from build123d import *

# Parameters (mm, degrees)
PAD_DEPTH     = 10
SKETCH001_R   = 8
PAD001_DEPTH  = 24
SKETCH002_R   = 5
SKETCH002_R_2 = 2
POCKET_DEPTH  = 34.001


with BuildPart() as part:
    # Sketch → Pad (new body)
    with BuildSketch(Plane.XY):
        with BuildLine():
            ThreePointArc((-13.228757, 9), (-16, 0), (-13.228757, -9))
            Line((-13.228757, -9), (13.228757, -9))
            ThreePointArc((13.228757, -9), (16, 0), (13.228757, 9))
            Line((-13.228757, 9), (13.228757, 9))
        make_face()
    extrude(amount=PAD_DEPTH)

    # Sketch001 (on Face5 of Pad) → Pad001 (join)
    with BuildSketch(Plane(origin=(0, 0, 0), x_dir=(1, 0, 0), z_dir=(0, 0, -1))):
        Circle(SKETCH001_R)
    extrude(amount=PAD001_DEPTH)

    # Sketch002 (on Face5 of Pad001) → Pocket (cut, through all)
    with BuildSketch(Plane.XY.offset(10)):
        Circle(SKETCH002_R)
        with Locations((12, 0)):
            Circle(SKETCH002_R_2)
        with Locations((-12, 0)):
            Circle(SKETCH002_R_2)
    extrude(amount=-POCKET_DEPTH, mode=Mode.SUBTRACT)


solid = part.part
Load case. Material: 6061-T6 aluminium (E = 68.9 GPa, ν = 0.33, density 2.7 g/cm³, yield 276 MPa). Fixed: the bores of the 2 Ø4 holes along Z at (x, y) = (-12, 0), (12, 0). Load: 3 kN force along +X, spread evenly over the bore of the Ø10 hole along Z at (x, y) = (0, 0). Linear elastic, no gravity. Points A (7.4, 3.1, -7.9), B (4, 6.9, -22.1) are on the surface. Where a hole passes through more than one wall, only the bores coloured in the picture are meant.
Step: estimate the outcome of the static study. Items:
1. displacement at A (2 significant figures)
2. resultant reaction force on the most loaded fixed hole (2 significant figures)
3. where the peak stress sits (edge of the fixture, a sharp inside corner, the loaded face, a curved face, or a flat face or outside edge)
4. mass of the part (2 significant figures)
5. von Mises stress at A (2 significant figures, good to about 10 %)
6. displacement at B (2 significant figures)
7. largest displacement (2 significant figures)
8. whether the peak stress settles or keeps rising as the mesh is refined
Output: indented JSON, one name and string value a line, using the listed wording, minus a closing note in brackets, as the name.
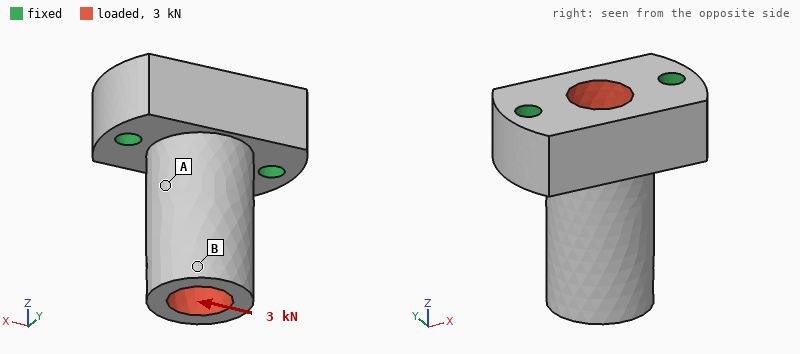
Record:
{
  "displacement at A": "21 µm",
  "resultant reaction force on the most loaded fixed hole": "2.3 kN",
  "where the peak stress sits": "a sharp inside corner",
  "mass of the part": "20 g",
  "von Mises stress at A": "29 MPa",
  "displacement at B": "46 µm",
  "largest displacement": "51 µm",
  "whether the peak stress settles or keeps rising as the mesh is refined": "keeps rising"
}
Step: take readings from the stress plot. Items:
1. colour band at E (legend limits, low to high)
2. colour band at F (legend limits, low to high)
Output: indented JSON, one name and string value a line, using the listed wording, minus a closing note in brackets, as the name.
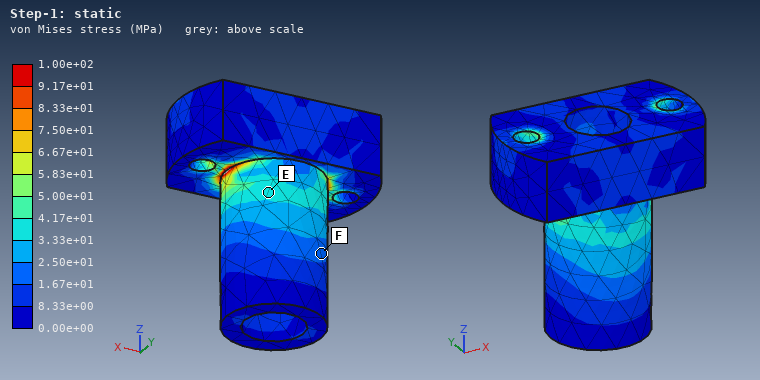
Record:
{
  "colour band at E": "3.33e+01 to 4.17e+01 MPa",
  "colour band at F": "1.67e+01 to 2.50e+01 MPa"
}
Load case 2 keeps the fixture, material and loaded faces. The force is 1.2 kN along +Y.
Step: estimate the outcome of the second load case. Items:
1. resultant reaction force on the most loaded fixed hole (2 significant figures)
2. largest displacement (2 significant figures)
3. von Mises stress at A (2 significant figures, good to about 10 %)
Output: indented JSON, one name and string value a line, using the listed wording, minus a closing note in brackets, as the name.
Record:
{
  "resultant reaction force on the most loaded fixed hole": "600 N",
  "largest displacement": "37 µm",
  "von Mises stress at A": "12 MPa"
}
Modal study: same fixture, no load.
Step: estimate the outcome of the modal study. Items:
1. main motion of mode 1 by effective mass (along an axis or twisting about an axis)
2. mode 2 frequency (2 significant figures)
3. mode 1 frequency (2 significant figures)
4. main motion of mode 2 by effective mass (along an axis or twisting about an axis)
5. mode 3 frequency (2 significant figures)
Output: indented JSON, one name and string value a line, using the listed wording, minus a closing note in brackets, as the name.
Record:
{
  "main motion of mode 1 by effective mass": "along Y",
  "mode 2 frequency": "14 kHz",
  "mode 1 frequency": "10 kHz",
  "main motion of mode 2 by effective mass": "along X",
  "mode 3 frequency": "29 kHz"
}
